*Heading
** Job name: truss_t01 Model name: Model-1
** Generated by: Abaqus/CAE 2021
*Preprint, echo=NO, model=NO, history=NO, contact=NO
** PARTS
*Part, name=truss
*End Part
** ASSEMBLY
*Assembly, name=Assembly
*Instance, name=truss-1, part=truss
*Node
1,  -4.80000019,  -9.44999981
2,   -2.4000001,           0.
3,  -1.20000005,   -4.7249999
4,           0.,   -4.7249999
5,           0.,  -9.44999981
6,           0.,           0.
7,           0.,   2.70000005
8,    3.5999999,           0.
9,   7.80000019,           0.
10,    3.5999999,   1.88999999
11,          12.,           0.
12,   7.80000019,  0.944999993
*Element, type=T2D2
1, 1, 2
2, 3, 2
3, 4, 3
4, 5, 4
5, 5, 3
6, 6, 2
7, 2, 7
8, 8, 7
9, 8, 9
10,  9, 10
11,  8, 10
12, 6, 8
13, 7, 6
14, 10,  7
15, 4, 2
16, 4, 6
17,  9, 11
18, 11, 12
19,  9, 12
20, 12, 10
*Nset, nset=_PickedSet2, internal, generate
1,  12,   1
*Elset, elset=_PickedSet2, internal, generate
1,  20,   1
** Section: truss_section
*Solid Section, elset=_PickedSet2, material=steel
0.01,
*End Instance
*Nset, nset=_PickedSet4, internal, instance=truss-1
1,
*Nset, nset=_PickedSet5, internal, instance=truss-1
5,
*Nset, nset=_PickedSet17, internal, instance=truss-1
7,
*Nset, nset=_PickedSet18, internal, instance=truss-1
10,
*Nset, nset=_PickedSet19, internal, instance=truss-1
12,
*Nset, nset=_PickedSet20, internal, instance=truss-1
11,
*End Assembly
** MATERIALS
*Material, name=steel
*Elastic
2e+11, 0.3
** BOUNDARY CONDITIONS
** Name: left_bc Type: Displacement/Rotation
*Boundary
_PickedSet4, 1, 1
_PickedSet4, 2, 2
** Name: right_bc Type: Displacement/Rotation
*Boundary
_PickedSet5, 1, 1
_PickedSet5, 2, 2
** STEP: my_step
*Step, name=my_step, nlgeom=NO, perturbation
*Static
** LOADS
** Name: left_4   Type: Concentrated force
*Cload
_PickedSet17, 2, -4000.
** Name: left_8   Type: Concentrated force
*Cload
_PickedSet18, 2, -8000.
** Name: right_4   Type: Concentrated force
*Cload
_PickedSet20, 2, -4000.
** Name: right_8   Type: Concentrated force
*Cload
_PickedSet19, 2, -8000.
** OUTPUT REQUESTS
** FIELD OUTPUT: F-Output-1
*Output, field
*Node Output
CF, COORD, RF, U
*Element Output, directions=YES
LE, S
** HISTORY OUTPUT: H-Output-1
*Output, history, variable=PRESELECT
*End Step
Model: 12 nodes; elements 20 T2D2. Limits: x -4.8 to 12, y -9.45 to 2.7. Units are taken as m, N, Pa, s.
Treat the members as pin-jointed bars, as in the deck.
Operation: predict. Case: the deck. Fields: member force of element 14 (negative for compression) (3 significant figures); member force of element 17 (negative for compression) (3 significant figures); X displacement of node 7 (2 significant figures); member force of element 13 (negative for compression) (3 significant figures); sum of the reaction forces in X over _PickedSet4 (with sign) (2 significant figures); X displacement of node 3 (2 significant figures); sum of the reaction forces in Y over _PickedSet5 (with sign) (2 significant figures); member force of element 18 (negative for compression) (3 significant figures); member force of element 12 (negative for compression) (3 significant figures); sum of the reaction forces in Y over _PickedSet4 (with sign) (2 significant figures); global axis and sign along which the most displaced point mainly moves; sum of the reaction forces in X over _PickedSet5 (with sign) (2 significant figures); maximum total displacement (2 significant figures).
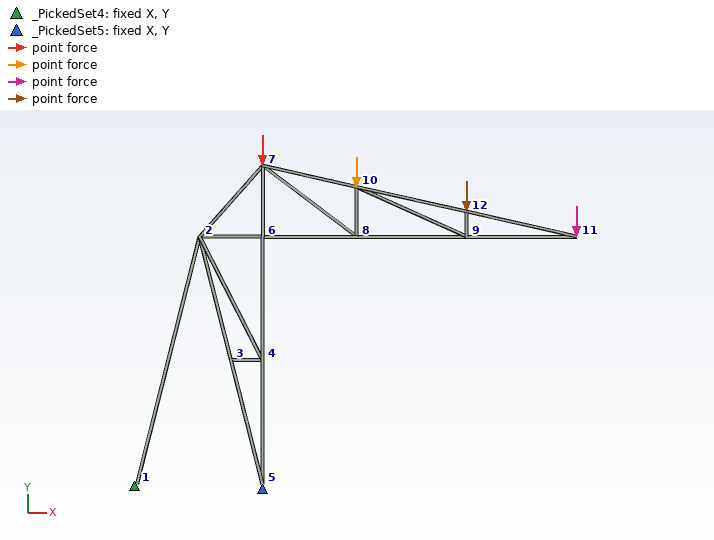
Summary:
36400 N
-17800 N
9.4e-04 m
-82000 N
-7400 N
-6.8e-04 m
53000 N
18200 N
-51600 N
-29000 N
-Y
7400 N
0.0065 m
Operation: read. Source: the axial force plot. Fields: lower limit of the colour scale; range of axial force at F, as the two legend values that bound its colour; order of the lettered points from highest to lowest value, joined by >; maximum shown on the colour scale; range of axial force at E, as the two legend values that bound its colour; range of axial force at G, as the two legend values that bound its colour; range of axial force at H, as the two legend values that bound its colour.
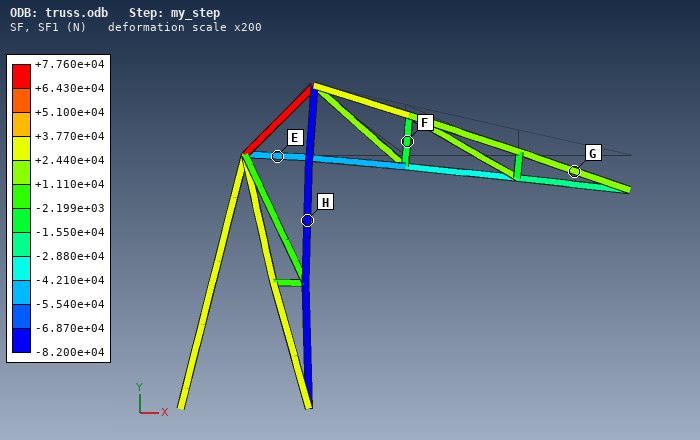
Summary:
-8.200e+04 N
-1.550e+04 to -2.199e+03 N
G > F > E > H
+7.760e+04 N
-5.540e+04 to -4.210e+04 N
+1.110e+04 to +2.440e+04 N
-8.200e+04 to -6.870e+04 N
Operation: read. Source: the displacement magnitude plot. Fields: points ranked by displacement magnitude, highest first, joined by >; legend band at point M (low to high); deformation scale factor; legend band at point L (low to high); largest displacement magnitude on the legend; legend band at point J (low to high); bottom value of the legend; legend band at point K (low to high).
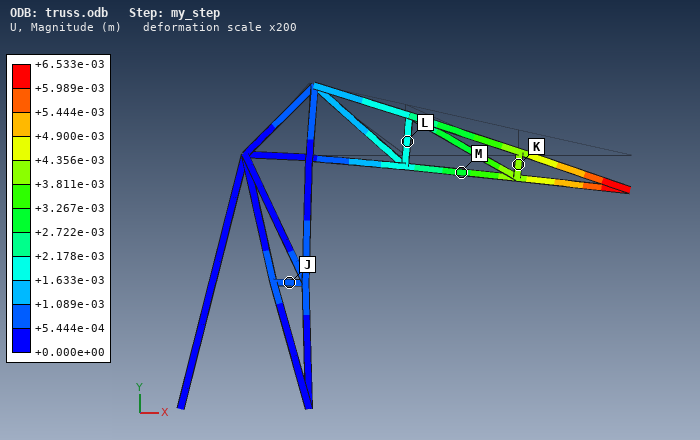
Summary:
K > M > L > J
+2.722e-03 to +3.267e-03 m
200
+1.633e-03 to +2.178e-03 m
+6.533e-03 m
+5.444e-04 to +1.089e-03 m
+0.000e+00 m
+3.811e-03 to +4.356e-03 m
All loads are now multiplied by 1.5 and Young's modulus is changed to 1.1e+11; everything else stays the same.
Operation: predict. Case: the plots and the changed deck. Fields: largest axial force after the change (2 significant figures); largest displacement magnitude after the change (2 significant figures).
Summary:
1.2e+05 N
0.018 m
